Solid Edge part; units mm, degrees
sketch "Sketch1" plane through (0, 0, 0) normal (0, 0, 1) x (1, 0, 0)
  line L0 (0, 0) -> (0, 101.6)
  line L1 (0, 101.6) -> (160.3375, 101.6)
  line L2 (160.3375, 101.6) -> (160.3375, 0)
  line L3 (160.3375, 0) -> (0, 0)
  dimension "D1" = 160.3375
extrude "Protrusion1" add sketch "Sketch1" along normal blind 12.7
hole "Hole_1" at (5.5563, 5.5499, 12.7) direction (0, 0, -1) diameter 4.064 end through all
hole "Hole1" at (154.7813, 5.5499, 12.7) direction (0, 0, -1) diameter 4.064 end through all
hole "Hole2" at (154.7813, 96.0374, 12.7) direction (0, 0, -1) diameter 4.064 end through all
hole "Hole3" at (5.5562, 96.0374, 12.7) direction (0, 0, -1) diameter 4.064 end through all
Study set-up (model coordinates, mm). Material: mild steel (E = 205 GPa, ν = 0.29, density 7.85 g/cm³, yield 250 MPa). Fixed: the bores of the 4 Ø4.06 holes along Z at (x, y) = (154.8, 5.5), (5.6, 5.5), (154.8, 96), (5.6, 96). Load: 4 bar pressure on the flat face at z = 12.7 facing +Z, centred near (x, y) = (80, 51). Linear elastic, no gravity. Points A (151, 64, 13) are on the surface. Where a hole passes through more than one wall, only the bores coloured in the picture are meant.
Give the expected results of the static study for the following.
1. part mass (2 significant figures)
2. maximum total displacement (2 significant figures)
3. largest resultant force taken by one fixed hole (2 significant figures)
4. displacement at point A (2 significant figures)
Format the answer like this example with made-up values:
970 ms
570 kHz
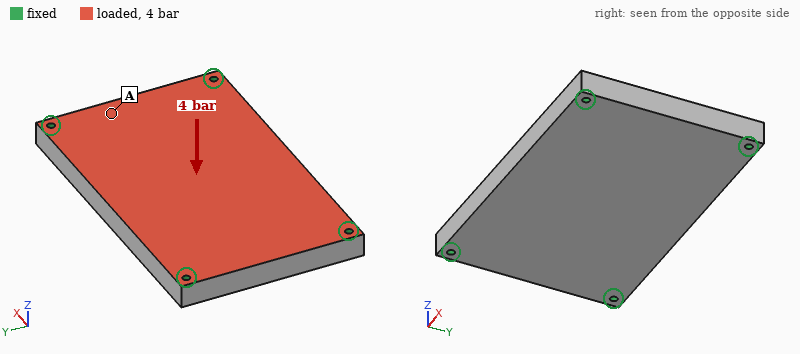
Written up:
1.6 kg
31 µm
1.6 kN
7.1 µm
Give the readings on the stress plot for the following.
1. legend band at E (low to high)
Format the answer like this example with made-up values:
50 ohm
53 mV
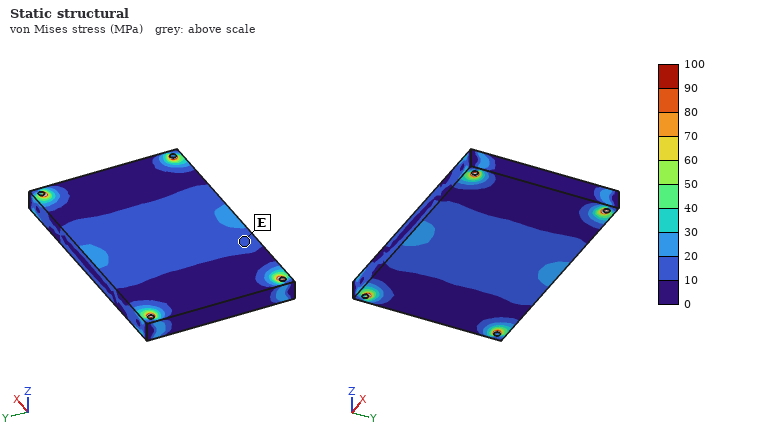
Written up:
10 to 20 MPa
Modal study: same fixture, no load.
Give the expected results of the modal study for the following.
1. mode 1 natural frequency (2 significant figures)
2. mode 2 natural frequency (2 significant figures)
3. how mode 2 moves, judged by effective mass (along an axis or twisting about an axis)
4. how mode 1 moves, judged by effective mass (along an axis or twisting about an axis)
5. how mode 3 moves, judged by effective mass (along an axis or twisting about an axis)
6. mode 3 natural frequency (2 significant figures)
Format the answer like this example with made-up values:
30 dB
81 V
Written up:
2100 Hz
3600 Hz
twisting about X
along Z
twisting about Y
5200 Hz
